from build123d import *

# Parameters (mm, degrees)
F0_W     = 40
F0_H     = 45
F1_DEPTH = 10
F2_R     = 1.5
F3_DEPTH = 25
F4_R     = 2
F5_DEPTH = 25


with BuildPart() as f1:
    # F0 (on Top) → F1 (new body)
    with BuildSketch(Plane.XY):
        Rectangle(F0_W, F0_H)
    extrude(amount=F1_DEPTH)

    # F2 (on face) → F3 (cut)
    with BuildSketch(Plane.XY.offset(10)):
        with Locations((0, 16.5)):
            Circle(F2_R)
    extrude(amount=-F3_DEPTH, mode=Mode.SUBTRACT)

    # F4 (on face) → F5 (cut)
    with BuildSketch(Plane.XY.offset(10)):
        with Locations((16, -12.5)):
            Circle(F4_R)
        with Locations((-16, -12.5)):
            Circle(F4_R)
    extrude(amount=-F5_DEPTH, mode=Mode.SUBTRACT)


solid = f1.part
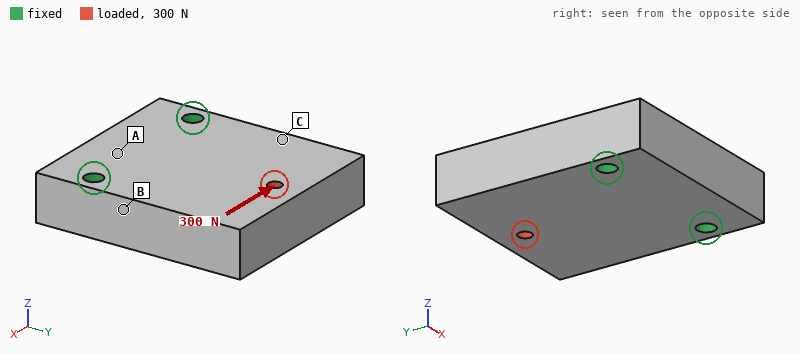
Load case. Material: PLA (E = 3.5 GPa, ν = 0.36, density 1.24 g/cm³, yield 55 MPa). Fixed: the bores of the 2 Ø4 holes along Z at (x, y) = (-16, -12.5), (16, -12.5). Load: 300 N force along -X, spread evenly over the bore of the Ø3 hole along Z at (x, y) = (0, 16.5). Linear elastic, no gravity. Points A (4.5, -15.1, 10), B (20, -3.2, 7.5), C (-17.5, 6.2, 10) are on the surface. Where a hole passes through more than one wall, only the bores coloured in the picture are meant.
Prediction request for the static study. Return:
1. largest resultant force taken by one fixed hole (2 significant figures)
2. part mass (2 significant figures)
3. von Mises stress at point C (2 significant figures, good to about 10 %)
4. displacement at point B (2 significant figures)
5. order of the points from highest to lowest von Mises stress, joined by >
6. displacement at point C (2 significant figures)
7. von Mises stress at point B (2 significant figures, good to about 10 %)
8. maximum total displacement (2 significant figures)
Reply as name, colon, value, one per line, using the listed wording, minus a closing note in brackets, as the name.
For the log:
largest resultant force taken by one fixed hole: 300 N
part mass: 22 g
von Mises stress at point C: 1.1 MPa
displacement at point B: 13 µm
order of the points from highest to lowest von Mises stress, joined by >: B > C > A
displacement at point C: 22 µm
von Mises stress at point B: 2.1 MPa
maximum total displacement: 39 µm
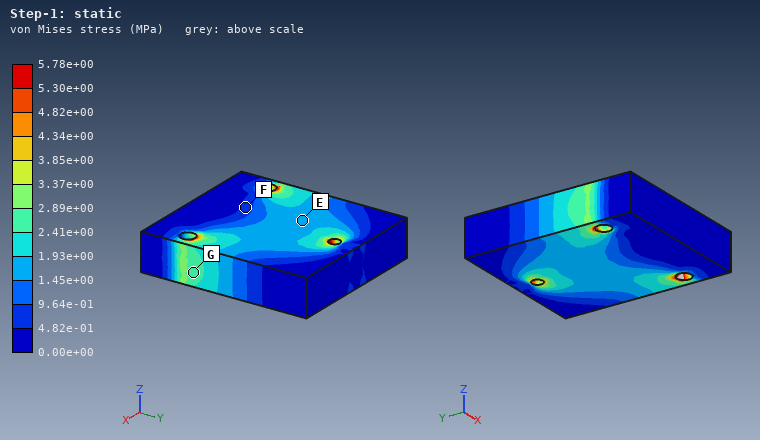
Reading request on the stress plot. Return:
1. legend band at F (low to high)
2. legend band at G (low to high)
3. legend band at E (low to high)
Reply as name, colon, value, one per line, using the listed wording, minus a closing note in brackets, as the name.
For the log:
legend band at F: 4.82e-01 to 9.64e-01 MPa
legend band at G: 2.41e+00 to 2.89e+00 MPa
legend band at E: 1.45e+00 to 1.93e+00 MPa
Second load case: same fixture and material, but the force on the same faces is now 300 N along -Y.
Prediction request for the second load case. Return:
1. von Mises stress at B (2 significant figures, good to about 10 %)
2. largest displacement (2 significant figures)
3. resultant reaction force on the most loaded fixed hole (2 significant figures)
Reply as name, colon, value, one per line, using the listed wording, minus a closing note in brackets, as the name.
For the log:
von Mises stress at B: 0.78 MPa
largest displacement: 16 µm
resultant reaction force on the most loaded fixed hole: 150 N
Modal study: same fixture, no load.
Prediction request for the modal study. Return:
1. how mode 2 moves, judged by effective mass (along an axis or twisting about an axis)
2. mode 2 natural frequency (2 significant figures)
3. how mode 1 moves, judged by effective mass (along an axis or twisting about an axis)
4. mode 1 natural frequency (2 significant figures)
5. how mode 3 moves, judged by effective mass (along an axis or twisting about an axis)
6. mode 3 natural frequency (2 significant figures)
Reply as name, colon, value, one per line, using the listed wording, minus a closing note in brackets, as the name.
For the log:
how mode 2 moves, judged by effective mass: twisting about Y
mode 2 natural frequency: 4100 Hz
how mode 1 moves, judged by effective mass: along Z
mode 1 natural frequency: 1800 Hz
how mode 3 moves, judged by effective mass: along X
mode 3 natural frequency: 5200 Hz
